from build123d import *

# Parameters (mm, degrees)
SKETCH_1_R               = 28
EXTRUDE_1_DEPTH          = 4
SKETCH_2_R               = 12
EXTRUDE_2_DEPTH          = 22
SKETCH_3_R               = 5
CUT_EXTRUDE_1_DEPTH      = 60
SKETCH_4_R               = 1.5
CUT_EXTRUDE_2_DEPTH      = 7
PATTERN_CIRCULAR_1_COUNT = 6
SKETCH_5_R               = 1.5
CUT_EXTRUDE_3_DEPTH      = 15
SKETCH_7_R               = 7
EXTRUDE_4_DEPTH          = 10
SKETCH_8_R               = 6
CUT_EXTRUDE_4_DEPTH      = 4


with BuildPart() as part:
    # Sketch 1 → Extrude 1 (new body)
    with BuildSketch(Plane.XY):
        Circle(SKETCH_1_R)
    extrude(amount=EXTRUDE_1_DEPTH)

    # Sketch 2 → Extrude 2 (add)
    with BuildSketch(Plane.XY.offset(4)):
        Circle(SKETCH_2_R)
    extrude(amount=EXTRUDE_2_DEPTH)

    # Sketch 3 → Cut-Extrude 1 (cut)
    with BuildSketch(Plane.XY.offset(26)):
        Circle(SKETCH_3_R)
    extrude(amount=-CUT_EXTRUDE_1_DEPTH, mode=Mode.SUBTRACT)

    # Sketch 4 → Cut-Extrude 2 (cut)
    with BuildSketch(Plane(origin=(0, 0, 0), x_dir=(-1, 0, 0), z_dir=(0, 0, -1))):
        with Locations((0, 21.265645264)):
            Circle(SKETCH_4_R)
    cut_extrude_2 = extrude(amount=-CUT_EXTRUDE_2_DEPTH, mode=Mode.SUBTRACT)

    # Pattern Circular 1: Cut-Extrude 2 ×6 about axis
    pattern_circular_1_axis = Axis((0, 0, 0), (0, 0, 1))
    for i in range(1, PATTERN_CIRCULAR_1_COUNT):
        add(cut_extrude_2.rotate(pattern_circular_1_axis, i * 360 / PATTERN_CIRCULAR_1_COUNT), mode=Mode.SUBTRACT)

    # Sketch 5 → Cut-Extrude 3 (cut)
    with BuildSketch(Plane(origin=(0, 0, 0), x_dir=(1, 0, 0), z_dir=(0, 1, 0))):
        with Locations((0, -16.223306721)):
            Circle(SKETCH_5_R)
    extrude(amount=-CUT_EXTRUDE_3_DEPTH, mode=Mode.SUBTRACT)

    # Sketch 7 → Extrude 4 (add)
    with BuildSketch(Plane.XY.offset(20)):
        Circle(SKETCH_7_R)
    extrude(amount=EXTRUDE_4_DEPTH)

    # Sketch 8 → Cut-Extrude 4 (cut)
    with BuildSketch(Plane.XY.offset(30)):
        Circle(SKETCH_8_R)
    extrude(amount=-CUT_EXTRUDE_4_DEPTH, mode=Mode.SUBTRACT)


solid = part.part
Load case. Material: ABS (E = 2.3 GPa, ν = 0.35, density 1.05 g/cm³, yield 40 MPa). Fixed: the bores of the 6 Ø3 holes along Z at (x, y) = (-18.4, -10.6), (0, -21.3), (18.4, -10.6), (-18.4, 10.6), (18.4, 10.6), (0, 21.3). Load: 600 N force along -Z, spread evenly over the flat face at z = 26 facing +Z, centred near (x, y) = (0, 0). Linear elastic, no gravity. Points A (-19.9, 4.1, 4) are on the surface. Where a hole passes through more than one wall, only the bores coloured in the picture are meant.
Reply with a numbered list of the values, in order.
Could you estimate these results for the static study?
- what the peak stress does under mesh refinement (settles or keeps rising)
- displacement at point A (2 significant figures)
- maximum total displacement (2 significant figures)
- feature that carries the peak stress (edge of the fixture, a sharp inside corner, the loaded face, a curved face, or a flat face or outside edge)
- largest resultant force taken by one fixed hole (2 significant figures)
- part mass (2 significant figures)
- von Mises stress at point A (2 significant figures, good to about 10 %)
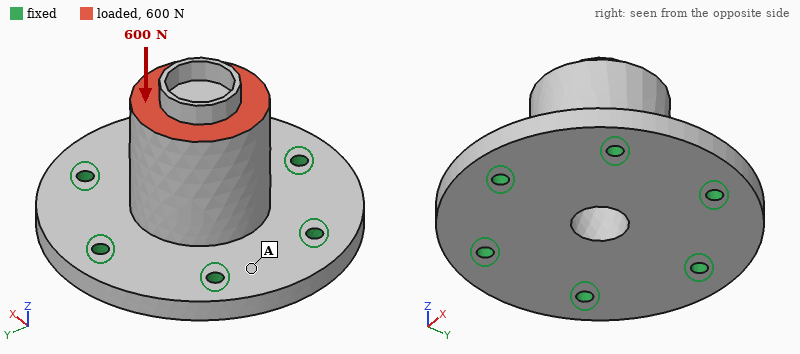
1. keeps rising
2. 0.019 mm
3. 0.11 mm
4. edge of the fixture
5. 110 N
6. 19 g
7. 3.0 MPa
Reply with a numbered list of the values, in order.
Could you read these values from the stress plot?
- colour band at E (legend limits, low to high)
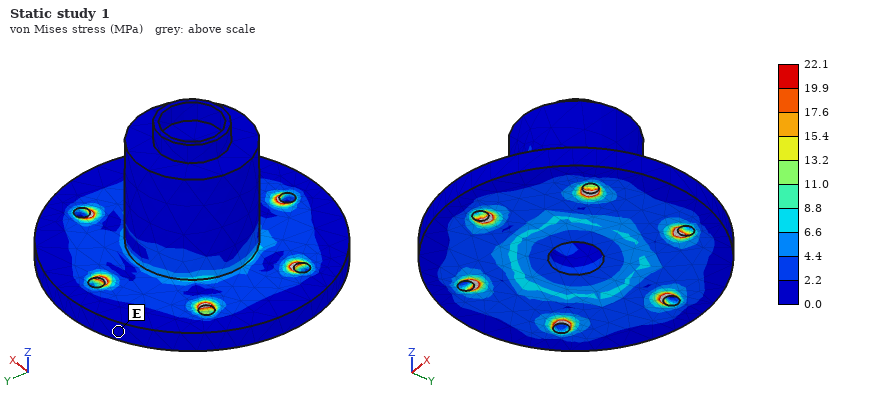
1. 0.0 to 2.2 MPa
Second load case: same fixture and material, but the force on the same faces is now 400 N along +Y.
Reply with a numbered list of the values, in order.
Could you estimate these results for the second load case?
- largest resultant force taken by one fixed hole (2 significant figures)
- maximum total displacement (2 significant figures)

1. 210 N
2. 0.38 mm
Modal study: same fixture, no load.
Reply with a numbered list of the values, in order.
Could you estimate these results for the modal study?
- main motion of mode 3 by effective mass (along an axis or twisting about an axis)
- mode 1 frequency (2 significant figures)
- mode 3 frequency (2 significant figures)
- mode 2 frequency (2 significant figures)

1. along Z
2. 2700 Hz
3. 3600 Hz
4. 2700 Hz
